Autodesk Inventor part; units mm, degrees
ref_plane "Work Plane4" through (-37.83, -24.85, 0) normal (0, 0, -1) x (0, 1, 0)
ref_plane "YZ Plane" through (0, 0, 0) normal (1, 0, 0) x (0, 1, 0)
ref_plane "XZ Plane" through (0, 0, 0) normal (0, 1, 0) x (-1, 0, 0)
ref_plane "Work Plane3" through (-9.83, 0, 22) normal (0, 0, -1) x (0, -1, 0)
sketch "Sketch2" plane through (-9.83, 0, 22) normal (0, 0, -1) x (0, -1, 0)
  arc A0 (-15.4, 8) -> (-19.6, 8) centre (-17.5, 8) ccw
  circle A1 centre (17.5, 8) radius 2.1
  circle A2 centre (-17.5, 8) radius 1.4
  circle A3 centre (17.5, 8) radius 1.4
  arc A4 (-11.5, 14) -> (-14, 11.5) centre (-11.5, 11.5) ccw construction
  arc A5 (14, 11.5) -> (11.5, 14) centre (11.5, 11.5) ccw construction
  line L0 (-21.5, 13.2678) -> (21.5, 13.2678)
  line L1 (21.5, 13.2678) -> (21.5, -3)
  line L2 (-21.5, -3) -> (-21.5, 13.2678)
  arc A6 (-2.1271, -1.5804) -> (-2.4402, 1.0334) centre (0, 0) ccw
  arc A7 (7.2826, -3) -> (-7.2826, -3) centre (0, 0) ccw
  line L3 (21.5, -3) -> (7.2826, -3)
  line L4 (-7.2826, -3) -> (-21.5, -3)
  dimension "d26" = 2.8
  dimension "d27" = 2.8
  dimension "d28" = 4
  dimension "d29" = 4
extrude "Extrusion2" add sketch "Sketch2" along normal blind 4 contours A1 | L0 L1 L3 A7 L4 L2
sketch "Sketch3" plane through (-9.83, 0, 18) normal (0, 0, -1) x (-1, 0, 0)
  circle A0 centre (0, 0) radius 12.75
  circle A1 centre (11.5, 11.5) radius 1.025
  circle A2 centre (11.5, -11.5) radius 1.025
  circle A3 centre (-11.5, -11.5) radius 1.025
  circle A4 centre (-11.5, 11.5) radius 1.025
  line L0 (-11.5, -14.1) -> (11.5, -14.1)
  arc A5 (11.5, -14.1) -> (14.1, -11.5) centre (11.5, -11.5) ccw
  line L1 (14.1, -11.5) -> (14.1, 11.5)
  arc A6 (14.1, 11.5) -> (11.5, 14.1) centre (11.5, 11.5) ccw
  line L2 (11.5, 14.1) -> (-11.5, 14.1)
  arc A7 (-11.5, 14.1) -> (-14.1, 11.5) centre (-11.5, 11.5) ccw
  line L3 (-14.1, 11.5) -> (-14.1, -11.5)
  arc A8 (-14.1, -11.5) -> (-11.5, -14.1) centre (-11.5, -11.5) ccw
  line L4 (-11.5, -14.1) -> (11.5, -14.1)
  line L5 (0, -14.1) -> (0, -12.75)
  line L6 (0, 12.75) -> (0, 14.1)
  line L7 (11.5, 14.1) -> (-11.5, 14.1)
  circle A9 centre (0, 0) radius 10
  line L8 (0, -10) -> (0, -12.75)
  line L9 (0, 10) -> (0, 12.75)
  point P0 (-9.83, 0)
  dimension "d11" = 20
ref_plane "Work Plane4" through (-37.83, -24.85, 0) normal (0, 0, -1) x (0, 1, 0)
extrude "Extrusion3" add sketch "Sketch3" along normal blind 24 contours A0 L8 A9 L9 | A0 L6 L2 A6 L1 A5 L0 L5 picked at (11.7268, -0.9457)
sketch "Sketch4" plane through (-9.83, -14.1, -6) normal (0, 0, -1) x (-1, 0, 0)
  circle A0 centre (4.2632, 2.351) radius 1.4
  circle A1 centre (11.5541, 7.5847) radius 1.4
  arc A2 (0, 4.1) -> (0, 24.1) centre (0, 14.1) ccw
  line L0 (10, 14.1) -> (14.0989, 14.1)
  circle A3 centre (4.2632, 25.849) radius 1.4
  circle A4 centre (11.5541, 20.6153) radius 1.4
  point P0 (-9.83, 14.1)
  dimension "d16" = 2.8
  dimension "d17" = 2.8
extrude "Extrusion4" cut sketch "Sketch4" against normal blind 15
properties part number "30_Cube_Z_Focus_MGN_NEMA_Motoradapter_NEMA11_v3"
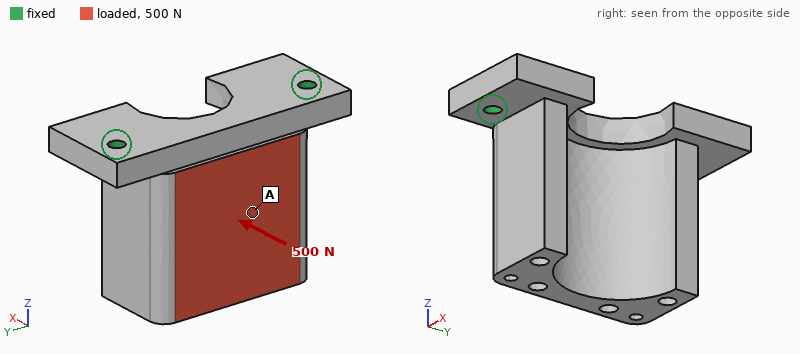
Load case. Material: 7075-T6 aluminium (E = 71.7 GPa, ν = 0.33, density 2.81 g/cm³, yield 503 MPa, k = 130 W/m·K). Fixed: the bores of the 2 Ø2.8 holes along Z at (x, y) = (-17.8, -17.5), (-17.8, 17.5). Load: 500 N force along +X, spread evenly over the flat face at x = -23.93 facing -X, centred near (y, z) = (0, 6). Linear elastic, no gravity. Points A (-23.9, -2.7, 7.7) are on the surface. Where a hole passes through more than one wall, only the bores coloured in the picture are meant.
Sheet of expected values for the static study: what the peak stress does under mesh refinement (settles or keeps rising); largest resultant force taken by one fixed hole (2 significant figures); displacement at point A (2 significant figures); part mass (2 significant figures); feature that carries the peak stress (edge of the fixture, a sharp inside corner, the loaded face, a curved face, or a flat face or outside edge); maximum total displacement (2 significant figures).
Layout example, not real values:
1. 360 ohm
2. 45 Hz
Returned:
1. keeps rising
2. 290 N
3. 42 µm
4. 21 g
5. edge of the fixture
6. 77 µm
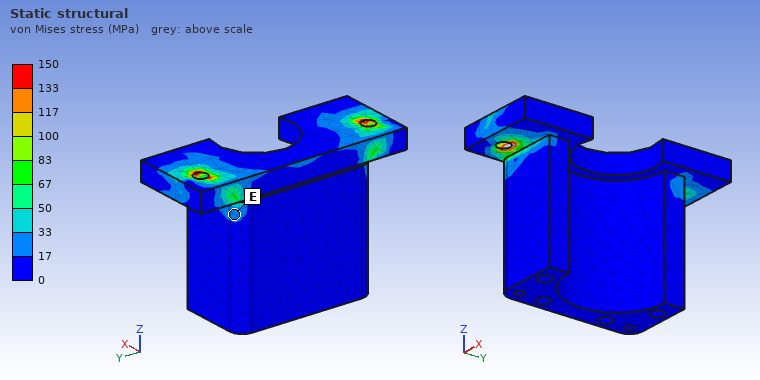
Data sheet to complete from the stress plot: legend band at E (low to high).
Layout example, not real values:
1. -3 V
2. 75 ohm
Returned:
1. 17 to 33 MPa
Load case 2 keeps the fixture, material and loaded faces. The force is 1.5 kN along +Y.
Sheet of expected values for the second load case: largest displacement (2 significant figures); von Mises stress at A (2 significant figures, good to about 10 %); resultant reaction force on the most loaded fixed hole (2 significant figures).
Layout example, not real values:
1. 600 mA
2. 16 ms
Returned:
1. 19 µm
2. 19 MPa
3. 1.0 kN
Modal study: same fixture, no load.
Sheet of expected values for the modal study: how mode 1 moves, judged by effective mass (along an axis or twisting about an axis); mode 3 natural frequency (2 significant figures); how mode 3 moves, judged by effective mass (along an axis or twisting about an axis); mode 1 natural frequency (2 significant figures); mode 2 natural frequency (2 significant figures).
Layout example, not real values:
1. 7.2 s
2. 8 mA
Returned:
1. along X
2. 14 kHz
3. along Y
4. 4200 Hz
5. 9900 Hz
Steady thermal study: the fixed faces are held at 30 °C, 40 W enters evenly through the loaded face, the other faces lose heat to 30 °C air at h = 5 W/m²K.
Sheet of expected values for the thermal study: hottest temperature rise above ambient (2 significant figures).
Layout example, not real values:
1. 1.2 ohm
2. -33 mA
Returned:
1. 42 K
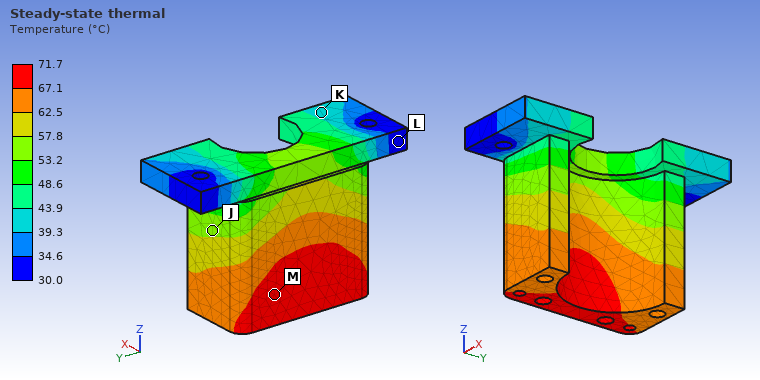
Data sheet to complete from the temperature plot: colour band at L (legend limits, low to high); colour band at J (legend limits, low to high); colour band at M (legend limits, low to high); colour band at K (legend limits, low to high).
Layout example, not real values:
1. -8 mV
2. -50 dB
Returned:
1. 30.0 to 34.6 °C
2. 53.2 to 57.8 °C
3. 67.1 to 71.7 °C
4. 39.3 to 43.9 °C
